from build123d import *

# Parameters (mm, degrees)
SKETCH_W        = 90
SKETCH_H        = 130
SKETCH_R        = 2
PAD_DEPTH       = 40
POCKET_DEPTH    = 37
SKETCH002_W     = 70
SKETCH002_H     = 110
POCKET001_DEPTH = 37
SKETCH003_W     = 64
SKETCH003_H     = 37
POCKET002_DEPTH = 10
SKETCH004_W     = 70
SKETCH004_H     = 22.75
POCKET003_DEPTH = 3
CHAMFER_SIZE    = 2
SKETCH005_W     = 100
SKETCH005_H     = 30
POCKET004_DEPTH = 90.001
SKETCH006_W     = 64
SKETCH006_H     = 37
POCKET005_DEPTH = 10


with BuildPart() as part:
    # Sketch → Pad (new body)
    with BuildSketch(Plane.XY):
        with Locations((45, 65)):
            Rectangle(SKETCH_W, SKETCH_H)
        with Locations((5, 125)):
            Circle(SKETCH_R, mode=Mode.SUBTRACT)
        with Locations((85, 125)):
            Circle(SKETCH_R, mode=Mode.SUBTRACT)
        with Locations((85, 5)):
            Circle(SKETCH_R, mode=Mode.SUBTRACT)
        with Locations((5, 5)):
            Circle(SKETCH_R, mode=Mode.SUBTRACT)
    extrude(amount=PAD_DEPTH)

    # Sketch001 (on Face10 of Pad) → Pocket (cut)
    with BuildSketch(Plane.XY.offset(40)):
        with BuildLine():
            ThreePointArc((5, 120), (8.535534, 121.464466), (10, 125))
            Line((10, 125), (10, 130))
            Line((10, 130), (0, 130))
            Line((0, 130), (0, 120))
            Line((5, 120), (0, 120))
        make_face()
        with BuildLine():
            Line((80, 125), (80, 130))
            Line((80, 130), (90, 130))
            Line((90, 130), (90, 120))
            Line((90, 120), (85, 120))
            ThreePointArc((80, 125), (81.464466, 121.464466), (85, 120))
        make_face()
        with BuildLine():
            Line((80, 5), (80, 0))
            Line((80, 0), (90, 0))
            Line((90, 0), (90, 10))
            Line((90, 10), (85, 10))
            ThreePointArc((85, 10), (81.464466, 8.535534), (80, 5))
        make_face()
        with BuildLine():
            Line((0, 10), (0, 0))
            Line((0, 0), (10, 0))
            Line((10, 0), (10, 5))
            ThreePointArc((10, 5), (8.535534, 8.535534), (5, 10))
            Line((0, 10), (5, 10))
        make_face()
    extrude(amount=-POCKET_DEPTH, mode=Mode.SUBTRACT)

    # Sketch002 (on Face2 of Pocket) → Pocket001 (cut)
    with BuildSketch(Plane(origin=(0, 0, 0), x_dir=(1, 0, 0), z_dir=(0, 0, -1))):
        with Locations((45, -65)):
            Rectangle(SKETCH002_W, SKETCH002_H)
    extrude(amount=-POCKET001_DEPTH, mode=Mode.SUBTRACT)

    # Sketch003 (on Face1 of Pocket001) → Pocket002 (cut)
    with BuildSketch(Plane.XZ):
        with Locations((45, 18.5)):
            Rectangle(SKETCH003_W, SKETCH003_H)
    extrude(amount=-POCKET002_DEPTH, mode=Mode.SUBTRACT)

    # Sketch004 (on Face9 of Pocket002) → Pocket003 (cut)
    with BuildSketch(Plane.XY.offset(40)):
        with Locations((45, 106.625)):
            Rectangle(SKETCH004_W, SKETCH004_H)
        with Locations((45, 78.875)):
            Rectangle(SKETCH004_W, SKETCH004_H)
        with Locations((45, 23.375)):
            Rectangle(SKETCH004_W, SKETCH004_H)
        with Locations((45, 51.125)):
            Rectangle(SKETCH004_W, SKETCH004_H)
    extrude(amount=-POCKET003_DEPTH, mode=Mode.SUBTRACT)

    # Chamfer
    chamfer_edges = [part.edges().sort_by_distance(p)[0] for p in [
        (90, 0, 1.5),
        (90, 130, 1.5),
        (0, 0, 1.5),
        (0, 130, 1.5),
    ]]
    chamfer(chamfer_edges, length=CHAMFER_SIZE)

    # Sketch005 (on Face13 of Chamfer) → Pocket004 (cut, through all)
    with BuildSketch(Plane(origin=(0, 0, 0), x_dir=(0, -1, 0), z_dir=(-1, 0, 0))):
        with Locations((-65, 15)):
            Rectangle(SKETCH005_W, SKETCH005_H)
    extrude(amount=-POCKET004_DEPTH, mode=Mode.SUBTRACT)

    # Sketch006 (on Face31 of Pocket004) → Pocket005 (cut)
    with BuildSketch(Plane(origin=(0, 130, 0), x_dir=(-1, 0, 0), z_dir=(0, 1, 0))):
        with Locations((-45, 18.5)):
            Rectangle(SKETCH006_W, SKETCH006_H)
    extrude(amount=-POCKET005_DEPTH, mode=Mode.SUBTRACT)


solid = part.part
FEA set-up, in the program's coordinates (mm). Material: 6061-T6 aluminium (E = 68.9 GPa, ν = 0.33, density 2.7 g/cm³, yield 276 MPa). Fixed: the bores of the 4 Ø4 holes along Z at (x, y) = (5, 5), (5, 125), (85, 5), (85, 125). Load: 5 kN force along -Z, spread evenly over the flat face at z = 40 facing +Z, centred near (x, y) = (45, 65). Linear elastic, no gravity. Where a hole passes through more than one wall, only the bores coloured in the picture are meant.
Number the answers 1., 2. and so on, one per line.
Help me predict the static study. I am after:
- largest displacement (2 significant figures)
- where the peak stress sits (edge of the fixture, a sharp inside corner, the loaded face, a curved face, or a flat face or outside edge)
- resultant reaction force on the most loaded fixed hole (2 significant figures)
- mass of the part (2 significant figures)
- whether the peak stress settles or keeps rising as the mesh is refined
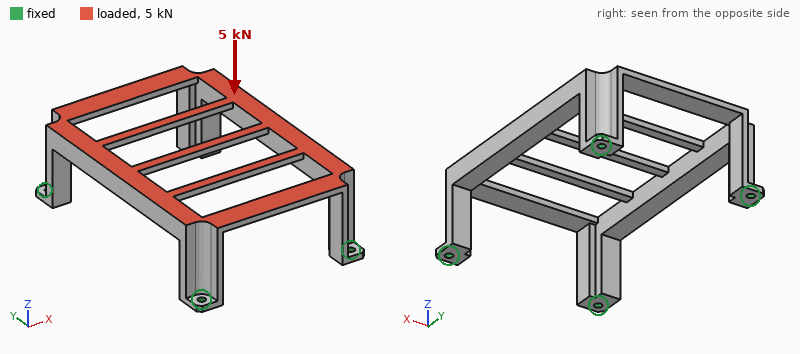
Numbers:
1. 0.80 mm
2. edge of the fixture
3. 1.4 kN
4. 110 g
5. keeps rising
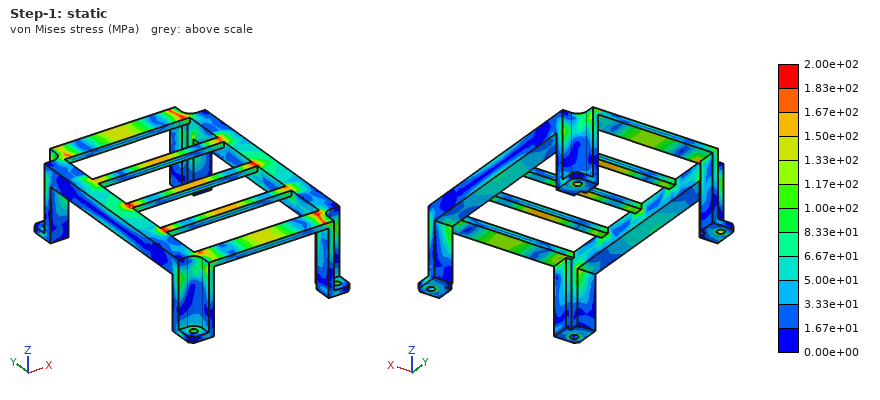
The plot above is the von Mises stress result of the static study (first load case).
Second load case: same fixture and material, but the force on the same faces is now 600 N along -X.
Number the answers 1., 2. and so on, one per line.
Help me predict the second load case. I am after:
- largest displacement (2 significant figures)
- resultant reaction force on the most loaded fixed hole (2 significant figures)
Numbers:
1. 0.20 mm
2. 160 N
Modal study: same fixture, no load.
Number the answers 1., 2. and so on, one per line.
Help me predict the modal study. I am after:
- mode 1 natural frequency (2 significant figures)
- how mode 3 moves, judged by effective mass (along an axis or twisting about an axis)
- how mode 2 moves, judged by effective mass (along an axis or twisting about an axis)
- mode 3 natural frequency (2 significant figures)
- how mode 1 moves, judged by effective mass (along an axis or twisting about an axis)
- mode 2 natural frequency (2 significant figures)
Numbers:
1. 1000 Hz
2. twisting about Z
3. along Y
4. 1900 Hz
5. along X
6. 1700 Hz
